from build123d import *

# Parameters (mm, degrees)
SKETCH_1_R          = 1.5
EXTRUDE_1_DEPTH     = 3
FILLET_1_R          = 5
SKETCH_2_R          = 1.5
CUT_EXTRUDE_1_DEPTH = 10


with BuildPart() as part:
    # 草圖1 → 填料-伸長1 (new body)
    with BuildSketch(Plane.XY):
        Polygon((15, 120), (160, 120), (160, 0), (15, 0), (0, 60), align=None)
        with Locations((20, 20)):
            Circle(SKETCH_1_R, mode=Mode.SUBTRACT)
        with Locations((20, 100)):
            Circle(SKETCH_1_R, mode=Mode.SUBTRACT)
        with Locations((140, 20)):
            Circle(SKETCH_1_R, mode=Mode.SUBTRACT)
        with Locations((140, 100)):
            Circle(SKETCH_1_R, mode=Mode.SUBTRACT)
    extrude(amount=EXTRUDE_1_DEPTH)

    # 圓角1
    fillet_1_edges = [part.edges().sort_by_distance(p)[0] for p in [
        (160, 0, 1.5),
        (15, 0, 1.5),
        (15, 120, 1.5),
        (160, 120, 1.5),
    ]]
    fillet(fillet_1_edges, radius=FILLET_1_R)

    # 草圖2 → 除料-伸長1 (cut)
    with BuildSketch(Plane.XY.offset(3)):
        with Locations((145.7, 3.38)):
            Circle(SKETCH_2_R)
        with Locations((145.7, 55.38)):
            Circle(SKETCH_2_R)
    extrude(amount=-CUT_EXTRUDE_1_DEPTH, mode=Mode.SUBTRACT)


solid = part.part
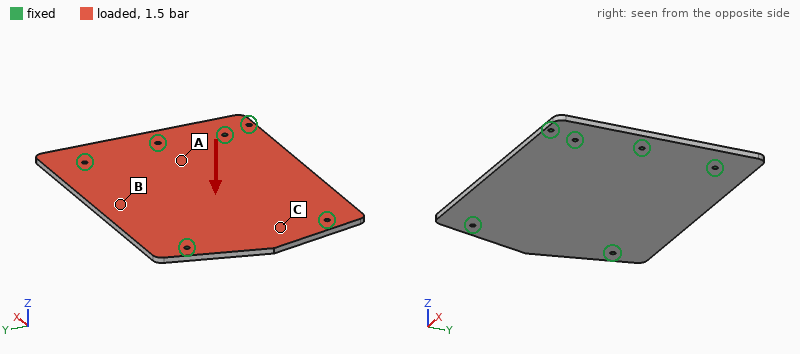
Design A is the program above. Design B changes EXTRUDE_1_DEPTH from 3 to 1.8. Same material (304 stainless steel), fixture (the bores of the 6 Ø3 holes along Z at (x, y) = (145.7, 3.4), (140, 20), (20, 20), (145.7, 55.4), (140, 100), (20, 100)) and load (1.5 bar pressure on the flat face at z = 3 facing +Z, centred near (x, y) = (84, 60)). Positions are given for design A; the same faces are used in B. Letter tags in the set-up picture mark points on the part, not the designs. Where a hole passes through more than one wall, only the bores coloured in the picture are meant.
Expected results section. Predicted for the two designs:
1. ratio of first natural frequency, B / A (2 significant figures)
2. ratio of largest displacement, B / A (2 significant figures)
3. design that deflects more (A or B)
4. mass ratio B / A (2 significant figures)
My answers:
0.62
4.4
B
0.60
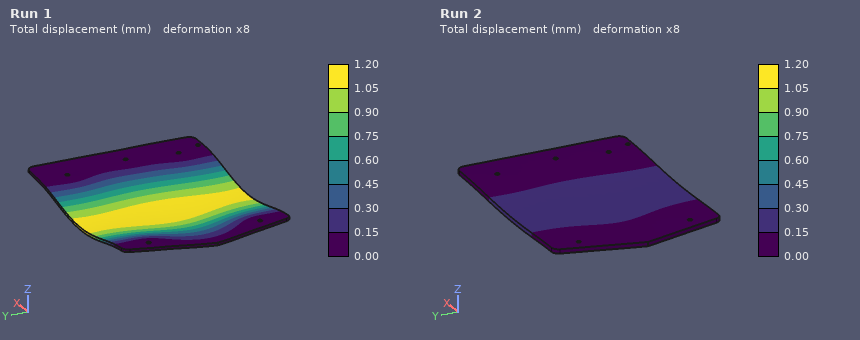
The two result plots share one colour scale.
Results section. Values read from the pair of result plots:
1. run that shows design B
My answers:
Run 1
